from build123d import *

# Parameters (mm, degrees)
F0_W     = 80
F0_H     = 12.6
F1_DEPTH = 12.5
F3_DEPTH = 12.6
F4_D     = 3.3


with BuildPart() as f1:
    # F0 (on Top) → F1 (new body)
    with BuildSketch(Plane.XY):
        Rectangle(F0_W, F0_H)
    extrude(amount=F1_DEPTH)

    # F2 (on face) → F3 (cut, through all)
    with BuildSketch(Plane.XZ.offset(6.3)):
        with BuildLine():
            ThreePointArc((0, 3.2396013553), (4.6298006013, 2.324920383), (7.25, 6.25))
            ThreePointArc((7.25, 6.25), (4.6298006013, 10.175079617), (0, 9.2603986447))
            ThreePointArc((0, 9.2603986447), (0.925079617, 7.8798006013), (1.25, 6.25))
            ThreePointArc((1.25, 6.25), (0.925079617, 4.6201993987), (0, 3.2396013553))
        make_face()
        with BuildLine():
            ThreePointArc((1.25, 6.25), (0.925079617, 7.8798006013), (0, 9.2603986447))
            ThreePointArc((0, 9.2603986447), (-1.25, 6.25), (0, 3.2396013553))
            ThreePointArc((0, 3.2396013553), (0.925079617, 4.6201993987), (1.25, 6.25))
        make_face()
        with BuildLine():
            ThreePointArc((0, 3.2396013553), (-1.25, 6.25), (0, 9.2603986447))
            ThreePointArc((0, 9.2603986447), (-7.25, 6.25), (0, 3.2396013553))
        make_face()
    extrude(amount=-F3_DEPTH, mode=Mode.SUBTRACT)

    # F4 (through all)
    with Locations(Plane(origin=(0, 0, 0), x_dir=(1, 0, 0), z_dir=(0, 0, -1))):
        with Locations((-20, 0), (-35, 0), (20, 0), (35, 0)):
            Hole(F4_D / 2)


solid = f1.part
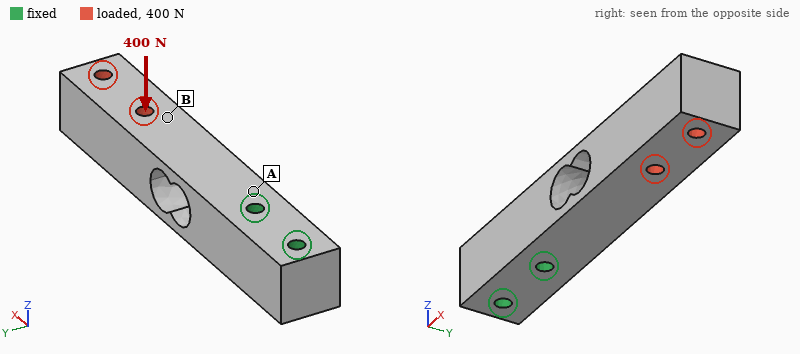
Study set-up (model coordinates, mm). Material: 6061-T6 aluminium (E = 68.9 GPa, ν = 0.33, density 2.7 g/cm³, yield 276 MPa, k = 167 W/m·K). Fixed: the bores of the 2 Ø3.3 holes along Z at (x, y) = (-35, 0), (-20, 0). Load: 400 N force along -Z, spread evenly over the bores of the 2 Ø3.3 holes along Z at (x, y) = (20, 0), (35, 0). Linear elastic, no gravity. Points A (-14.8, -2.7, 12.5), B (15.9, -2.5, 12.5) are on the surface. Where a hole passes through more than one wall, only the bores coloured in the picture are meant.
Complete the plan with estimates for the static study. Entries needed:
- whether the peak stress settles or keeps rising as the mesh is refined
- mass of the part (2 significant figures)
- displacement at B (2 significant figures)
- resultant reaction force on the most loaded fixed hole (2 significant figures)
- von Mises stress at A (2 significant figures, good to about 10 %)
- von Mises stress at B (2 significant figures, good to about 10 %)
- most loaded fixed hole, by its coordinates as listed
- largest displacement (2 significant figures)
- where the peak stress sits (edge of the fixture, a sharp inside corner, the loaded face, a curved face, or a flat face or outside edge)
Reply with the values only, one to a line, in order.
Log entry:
keeps rising
29 g
0.13 mm
610 N
53 MPa
15 MPa
(-20, 0)
0.22 mm
edge of the fixture
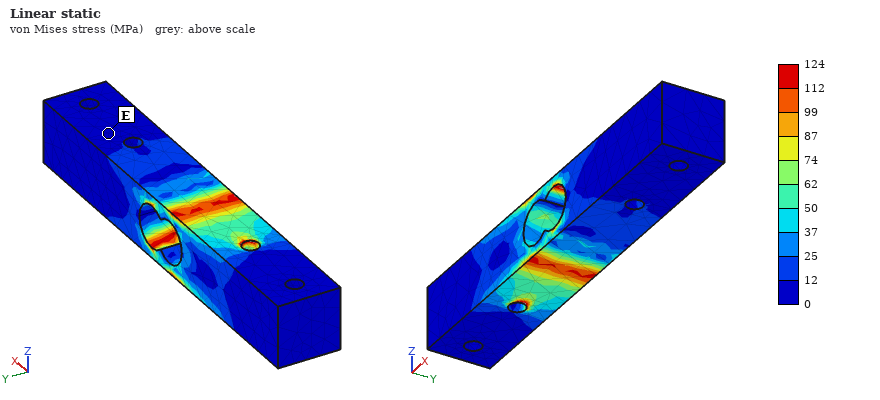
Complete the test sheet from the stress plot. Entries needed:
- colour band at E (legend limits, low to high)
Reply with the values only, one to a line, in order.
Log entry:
0 to 12 MPa
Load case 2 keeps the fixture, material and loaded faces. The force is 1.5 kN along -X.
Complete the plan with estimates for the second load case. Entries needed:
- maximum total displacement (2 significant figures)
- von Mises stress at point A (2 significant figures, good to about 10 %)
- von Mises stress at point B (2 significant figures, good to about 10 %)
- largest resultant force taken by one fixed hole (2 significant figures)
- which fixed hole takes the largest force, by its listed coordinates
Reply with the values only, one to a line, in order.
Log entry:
12 µm
12 MPa
12 MPa
1.3 kN
(-20, 0)
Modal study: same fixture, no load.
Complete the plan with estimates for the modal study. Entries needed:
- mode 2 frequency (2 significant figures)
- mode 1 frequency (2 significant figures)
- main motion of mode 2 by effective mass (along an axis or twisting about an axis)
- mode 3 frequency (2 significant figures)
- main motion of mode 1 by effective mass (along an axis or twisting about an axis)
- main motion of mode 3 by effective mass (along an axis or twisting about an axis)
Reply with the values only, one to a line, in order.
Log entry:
2200 Hz
2000 Hz
along Z
8200 Hz
along Y
twisting about X
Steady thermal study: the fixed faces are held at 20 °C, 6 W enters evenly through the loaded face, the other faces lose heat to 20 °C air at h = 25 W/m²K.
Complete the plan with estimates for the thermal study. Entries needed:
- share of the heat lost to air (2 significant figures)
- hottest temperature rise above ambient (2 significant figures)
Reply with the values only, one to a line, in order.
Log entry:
13 %
15 K
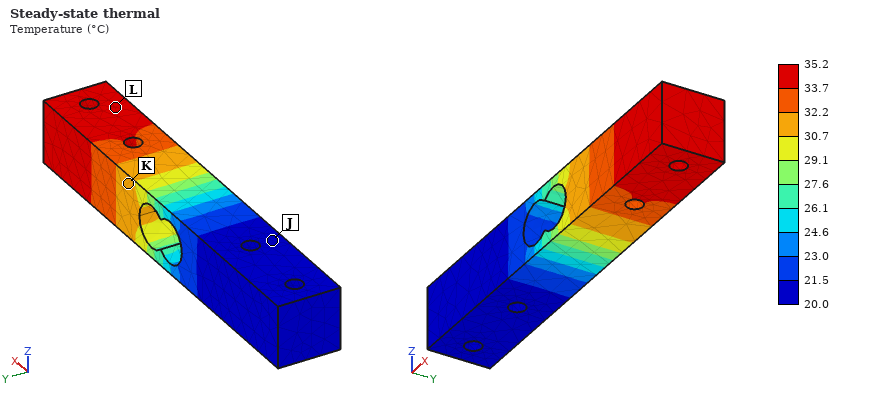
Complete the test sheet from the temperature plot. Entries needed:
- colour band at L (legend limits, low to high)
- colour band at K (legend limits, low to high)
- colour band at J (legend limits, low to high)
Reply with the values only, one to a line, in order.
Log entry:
33.7 to 35.2 °C
30.7 to 32.2 °C
20.0 to 21.5 °C
